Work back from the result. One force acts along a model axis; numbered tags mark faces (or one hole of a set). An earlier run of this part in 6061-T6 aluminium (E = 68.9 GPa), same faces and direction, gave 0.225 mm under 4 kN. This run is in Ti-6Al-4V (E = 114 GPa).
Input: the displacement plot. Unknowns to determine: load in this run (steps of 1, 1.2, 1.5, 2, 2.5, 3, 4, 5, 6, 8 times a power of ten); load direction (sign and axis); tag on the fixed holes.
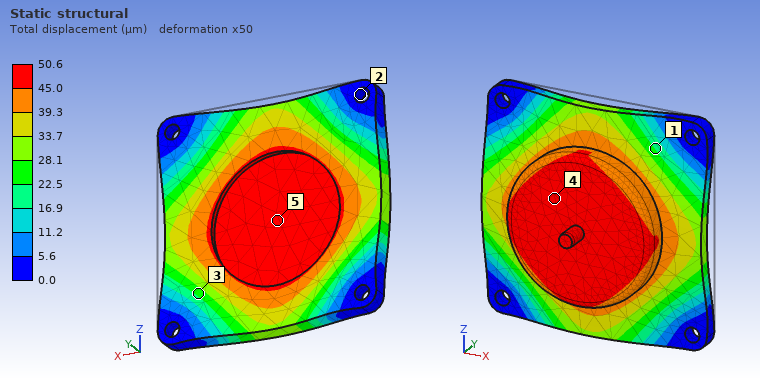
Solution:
1.5 kN
-Y
2
